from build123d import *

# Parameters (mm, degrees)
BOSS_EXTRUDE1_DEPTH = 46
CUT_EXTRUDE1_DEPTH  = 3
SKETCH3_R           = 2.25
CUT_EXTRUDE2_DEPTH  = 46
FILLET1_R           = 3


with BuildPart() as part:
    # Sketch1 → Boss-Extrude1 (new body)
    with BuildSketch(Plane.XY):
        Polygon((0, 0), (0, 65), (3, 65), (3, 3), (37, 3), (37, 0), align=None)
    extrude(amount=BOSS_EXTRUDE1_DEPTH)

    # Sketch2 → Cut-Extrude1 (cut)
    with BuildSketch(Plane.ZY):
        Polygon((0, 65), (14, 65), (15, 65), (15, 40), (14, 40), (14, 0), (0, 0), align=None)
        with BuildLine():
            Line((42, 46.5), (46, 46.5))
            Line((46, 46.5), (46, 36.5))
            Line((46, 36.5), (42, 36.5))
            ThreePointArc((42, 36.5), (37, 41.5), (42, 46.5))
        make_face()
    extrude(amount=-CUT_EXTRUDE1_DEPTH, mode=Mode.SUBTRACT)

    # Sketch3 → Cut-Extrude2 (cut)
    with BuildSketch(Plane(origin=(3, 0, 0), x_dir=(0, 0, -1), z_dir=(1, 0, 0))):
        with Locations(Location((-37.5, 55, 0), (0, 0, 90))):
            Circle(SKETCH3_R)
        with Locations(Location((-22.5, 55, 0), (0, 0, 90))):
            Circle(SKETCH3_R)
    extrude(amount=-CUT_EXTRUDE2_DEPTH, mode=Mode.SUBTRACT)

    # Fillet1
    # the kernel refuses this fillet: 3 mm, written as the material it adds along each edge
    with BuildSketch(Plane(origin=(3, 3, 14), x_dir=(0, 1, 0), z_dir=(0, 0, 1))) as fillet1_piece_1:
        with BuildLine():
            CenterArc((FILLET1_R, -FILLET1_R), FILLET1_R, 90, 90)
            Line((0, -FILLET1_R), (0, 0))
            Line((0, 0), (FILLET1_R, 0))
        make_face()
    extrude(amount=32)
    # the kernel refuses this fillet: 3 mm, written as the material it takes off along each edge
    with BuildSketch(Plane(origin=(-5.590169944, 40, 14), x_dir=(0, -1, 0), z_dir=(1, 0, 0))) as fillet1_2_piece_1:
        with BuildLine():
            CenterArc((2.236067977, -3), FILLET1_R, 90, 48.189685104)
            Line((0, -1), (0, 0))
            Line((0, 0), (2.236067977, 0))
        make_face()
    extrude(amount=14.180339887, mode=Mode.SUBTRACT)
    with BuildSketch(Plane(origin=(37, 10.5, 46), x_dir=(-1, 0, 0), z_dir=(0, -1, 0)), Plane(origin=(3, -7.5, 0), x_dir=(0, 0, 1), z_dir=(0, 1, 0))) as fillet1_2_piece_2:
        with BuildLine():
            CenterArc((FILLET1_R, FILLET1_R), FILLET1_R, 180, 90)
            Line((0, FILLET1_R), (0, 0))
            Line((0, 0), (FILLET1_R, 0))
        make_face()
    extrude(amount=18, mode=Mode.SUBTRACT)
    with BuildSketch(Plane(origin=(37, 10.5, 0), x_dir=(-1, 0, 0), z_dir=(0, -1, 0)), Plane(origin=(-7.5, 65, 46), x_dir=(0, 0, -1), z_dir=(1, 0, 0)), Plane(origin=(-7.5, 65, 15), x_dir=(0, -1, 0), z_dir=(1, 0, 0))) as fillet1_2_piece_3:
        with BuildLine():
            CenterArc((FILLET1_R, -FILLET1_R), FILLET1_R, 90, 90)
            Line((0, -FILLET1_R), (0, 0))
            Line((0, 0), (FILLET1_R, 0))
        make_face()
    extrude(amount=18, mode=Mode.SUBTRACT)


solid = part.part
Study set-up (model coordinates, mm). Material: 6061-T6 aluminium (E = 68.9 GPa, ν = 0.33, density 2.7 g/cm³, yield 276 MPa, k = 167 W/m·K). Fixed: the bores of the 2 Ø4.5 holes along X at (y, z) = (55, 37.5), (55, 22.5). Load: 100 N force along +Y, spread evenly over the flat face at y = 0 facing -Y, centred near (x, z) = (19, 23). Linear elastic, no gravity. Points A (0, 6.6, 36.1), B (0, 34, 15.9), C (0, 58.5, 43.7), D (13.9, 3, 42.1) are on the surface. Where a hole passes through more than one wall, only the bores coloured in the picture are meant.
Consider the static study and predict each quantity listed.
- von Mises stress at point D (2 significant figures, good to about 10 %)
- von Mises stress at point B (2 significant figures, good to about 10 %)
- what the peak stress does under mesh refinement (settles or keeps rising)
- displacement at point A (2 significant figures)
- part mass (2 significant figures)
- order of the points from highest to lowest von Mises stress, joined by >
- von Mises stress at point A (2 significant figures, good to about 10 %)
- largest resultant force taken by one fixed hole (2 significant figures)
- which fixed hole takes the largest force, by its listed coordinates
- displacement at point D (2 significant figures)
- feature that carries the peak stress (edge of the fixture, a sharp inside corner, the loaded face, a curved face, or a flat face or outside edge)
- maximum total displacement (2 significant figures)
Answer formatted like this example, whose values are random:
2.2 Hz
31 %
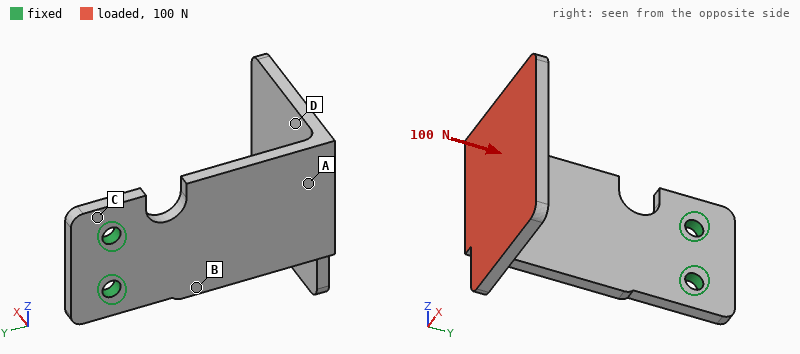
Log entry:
13 MPa
40 MPa
keeps rising
0.47 mm
28 g
B > A > D > C
29 MPa
88 N
(55, 22.5)
0.59 mm
edge of the fixture
1.0 mm
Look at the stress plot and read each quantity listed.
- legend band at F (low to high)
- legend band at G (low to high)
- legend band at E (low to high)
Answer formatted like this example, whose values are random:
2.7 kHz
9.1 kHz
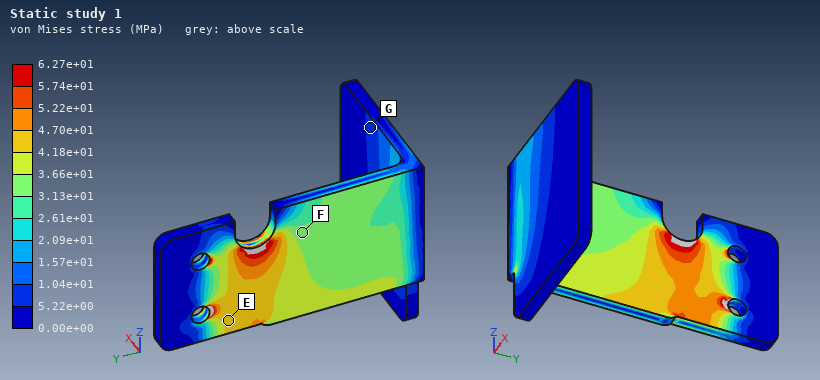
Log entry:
3.13e+01 to 3.66e+01 MPa
5.22e+00 to 1.04e+01 MPa
4.18e+01 to 4.70e+01 MPa
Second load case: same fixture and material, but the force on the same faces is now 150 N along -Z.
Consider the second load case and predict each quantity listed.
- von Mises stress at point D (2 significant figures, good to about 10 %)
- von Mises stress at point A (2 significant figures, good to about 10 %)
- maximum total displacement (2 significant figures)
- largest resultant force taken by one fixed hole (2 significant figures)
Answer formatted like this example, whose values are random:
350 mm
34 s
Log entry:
9.7 MPa
27 MPa
0.80 mm
510 N
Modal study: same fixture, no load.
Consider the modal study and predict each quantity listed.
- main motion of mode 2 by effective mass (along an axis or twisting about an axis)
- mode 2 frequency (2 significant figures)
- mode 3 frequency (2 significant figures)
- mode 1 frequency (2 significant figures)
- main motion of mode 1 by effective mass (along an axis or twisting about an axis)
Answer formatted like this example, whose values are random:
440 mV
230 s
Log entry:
along Z
660 Hz
1200 Hz
320 Hz
along X
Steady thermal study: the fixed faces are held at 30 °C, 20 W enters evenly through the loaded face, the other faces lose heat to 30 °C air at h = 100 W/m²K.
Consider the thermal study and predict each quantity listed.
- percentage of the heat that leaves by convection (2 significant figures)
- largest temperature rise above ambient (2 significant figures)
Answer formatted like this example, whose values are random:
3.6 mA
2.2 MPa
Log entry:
65 %
42 K
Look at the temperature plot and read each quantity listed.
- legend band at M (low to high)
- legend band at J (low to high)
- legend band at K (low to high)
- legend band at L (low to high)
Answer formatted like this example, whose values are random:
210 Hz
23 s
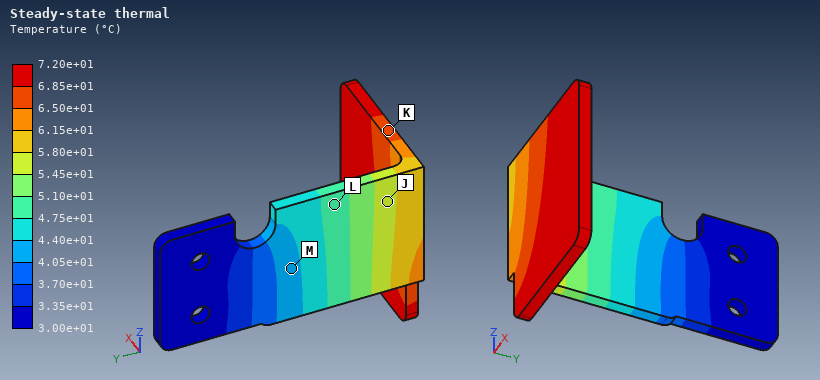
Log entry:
4.05e+01 to 4.40e+01 °C
5.45e+01 to 5.80e+01 °C
6.50e+01 to 6.85e+01 °C
4.75e+01 to 5.10e+01 °C
